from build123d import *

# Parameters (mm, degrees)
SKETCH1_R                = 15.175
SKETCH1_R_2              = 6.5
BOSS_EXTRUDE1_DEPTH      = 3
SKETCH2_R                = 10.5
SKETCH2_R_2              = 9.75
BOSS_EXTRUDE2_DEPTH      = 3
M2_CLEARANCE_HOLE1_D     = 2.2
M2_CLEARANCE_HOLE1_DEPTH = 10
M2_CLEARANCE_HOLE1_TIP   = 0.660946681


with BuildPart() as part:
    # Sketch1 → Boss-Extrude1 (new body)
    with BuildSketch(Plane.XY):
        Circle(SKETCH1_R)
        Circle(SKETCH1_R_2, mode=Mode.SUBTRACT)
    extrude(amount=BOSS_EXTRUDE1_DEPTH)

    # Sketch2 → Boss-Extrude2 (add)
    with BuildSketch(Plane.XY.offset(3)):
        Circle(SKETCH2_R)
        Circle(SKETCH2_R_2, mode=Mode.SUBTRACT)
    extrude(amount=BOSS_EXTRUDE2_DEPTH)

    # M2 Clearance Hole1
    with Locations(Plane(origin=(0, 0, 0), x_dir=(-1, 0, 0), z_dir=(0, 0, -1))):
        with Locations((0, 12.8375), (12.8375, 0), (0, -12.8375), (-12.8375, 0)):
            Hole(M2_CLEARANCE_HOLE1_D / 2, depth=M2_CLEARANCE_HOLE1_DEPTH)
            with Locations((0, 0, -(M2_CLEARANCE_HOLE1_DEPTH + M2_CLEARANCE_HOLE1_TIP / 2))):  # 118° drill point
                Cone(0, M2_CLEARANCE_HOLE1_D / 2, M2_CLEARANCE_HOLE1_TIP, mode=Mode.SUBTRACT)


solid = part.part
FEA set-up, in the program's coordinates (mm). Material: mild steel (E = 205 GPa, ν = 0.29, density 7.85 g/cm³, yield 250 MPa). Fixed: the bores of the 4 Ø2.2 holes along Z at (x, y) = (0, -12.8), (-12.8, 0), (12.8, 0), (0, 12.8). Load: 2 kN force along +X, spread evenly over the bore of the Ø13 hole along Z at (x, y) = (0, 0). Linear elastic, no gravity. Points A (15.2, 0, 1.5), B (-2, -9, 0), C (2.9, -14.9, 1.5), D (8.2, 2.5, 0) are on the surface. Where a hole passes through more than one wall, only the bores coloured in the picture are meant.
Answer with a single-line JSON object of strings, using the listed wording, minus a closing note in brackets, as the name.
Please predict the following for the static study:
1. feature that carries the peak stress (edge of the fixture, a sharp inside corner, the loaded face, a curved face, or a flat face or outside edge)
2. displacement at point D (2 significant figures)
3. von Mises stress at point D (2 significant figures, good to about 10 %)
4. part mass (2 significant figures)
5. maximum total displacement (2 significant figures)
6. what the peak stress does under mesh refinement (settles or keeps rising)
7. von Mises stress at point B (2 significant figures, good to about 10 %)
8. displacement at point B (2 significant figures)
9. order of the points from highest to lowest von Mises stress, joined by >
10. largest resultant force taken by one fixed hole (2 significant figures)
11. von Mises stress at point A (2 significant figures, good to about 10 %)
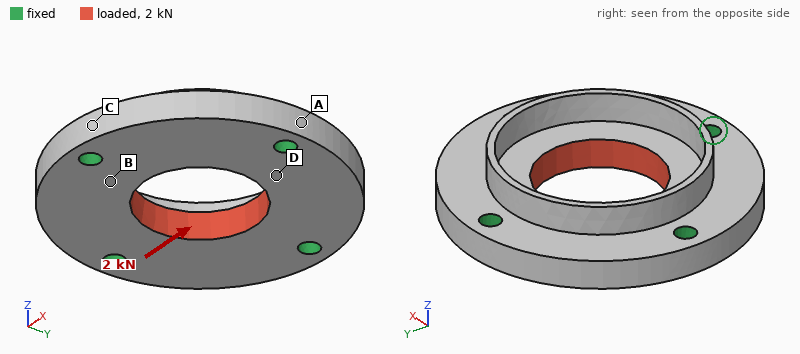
{"feature that carries the peak stress": "edge of the fixture", "displacement at point D": "0.74 µm", "von Mises stress at point D": "26 MPa", "part mass": "15 g", "maximum total displacement": "1.3 µm", "what the peak stress does under mesh refinement": "keeps rising", "von Mises stress at point B": "11 MPa", "displacement at point B": "0.75 µm", "order of the points from highest to lowest von Mises stress, joined by >": "D > A > B > C", "largest resultant force taken by one fixed hole": "550 N", "von Mises stress at point A": "20 MPa"}
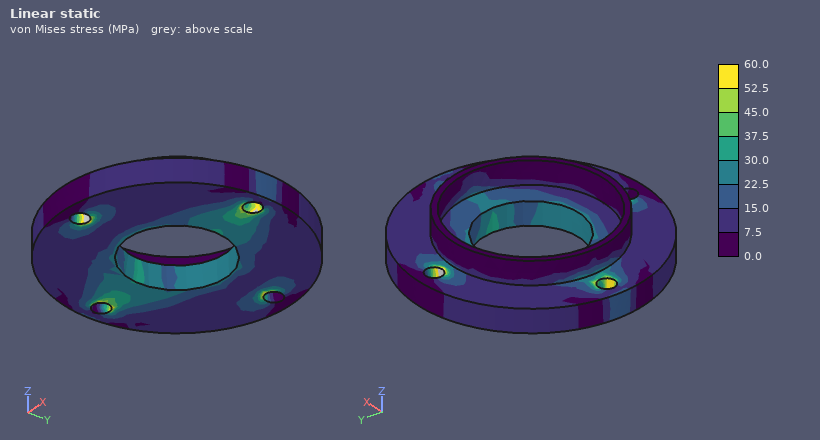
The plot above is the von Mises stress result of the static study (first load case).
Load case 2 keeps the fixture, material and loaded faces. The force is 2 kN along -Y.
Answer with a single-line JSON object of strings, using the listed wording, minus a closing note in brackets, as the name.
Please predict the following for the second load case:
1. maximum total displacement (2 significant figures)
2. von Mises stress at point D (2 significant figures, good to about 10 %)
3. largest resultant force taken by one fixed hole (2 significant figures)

{"maximum total displacement": "1.3 µm", "von Mises stress at point D": "12 MPa", "largest resultant force taken by one fixed hole": "550 N"}
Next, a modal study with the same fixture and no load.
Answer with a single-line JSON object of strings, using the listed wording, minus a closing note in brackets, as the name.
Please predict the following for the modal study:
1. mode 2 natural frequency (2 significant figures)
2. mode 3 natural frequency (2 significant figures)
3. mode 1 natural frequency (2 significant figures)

{"mode 2 natural frequency": "37 kHz", "mode 3 natural frequency": "37 kHz", "mode 1 natural frequency": "34 kHz"}
